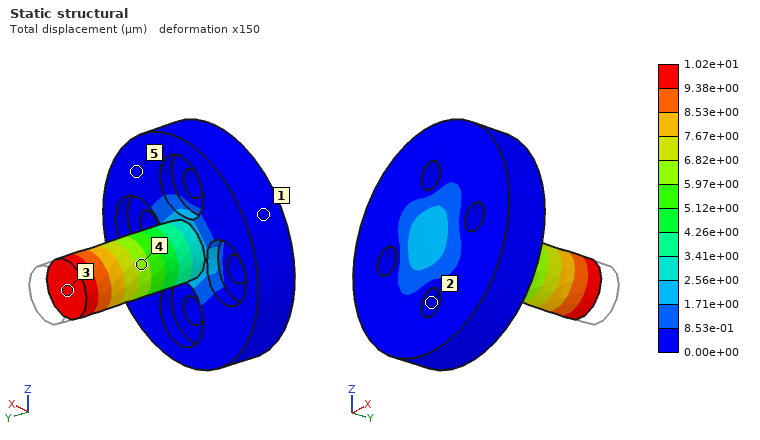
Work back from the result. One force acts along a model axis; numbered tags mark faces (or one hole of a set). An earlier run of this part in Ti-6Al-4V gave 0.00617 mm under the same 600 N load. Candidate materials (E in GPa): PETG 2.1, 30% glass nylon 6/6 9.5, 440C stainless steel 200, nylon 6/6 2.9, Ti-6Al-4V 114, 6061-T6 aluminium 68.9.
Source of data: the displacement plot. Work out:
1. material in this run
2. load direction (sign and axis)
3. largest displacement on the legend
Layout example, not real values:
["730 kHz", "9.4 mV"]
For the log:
["6061-T6 aluminium", "-Y", "1.02e+01 µm"]
